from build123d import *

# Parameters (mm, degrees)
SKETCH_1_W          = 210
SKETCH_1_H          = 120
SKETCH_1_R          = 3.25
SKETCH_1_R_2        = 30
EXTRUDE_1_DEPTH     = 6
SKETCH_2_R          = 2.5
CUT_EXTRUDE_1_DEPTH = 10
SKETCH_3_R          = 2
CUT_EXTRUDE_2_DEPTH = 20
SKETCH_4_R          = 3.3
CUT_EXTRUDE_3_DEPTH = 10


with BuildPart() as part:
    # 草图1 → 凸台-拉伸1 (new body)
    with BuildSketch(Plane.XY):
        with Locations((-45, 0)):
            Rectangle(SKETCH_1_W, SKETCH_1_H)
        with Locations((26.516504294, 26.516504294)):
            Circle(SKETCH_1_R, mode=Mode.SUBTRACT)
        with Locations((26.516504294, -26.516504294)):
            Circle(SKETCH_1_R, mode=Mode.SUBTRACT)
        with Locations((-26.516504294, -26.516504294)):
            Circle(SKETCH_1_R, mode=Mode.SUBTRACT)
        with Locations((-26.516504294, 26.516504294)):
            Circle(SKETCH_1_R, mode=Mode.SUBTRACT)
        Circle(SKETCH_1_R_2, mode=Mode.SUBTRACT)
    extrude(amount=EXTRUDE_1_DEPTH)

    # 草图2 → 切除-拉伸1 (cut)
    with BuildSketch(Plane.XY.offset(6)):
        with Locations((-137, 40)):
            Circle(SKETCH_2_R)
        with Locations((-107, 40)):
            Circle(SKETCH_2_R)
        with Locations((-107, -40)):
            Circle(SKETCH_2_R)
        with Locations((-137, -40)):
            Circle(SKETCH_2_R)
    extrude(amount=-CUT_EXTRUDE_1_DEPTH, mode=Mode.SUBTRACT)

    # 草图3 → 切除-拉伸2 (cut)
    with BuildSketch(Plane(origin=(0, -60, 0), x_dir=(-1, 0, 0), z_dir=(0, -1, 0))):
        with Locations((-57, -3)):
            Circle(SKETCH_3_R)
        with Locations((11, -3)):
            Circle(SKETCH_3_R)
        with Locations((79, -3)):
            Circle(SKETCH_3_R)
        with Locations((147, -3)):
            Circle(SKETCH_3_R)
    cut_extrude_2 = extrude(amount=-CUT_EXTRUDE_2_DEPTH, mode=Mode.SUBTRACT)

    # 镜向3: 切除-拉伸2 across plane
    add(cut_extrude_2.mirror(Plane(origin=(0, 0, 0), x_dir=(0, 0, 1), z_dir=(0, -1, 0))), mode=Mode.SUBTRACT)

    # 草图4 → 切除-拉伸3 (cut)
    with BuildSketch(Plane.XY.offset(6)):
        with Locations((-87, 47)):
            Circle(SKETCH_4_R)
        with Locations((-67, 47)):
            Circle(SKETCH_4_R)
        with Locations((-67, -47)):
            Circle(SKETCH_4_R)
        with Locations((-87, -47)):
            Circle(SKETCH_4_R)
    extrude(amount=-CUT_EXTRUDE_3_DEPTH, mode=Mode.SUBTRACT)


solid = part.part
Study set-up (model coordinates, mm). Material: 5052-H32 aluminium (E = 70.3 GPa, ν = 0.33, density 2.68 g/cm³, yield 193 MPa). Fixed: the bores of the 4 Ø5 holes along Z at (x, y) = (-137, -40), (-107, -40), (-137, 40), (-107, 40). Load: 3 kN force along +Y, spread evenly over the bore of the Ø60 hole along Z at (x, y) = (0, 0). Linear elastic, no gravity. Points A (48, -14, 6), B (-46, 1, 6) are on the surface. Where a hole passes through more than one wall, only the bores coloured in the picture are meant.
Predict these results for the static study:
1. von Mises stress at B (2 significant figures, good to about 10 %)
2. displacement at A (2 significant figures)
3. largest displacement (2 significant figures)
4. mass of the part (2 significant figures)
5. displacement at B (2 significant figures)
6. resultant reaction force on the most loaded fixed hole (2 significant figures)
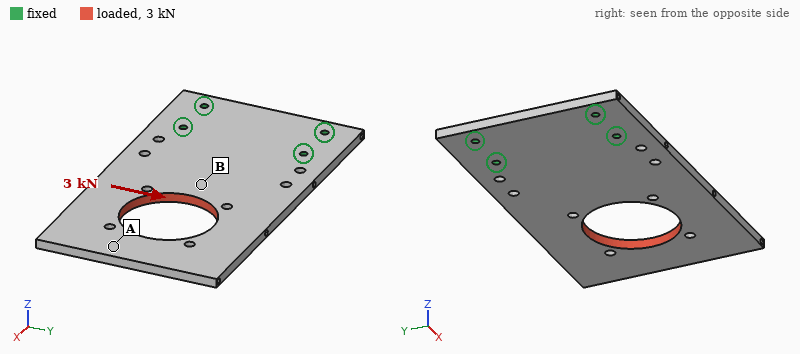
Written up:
18 MPa
0.10 mm
0.11 mm
350 g
0.027 mm
3.3 kN
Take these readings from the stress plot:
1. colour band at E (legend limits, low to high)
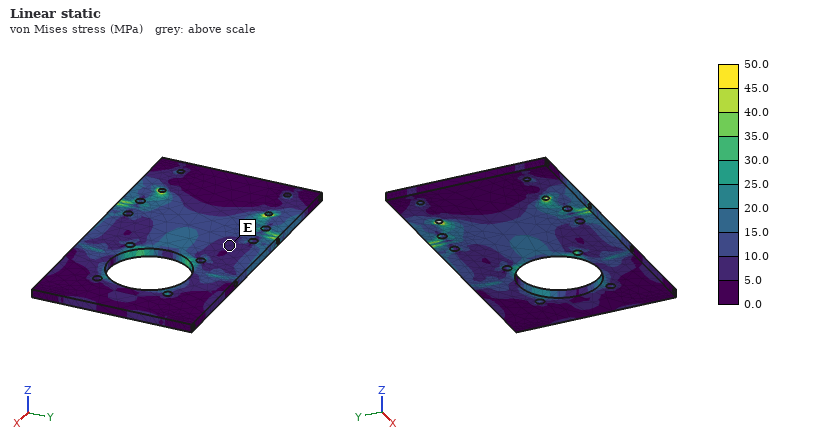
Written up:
5.0 to 10.0 MPa
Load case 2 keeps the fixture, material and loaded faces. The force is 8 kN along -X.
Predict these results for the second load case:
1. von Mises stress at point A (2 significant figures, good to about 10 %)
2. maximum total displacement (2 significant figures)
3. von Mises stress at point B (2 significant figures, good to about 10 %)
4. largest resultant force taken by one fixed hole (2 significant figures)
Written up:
9.3 MPa
45 µm
8.6 MPa
2.9 kN
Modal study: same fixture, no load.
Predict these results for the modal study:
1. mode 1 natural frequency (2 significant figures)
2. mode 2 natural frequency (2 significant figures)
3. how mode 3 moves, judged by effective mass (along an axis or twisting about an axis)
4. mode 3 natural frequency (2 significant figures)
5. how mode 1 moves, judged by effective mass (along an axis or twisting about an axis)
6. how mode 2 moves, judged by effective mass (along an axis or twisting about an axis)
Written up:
180 Hz
510 Hz
along Z
970 Hz
along Z
twisting about X
